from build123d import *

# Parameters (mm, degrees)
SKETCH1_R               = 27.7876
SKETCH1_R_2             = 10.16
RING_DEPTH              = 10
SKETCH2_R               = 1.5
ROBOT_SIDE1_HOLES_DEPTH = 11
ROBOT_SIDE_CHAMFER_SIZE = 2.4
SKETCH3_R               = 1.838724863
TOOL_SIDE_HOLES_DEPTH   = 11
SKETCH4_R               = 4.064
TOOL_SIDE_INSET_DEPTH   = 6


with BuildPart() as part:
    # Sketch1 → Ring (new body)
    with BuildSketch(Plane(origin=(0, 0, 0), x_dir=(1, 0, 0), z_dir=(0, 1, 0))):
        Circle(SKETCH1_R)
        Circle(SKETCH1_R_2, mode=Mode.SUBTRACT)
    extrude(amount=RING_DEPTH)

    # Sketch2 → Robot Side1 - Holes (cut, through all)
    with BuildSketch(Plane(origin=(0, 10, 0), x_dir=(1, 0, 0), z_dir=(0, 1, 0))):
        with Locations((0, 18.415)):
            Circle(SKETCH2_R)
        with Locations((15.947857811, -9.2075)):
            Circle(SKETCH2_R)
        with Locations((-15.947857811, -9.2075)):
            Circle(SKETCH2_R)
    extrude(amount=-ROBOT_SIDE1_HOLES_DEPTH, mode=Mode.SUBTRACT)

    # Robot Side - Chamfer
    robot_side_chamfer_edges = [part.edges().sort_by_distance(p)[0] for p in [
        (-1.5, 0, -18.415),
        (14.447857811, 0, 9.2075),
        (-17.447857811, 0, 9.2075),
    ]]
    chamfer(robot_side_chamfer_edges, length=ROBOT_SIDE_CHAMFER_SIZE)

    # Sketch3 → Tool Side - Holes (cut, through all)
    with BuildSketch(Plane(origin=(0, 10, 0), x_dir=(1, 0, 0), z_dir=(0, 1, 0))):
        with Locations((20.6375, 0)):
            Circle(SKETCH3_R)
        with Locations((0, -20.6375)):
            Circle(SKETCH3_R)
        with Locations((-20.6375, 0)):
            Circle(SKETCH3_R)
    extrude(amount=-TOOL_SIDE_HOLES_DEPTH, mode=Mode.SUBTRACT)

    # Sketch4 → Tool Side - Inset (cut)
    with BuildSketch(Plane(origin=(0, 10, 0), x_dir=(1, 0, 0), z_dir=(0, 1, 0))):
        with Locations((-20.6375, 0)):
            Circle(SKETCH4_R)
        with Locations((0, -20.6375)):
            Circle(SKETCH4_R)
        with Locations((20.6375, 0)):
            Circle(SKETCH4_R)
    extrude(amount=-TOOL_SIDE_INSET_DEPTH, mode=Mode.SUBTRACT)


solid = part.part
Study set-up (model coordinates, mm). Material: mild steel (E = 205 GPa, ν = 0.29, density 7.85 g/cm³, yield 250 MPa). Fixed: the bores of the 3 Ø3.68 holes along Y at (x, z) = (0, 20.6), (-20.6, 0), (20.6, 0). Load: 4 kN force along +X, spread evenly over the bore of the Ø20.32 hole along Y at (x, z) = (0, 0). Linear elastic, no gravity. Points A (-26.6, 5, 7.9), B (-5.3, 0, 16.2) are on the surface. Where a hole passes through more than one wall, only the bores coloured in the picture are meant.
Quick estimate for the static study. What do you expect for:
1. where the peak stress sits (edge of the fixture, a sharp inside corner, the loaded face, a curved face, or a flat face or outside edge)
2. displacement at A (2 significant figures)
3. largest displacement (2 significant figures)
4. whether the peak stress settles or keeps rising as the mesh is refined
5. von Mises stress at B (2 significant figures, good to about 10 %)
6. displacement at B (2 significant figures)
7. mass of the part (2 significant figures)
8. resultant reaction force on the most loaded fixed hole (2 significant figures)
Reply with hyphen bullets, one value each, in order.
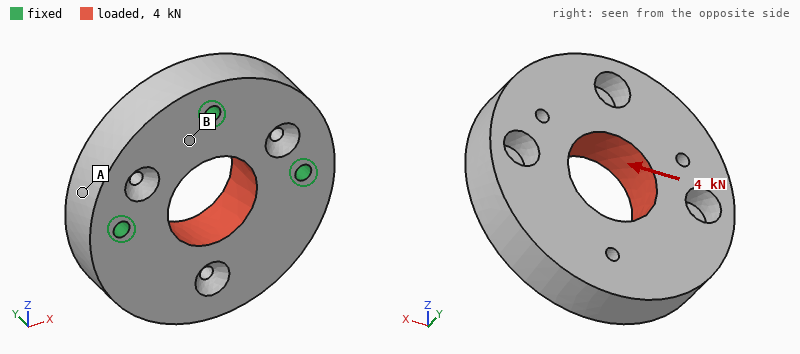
- edge of the fixture
- 1.3 µm
- 2.3 µm
- keeps rising
- 12 MPa
- 0.48 µm
- 150 g
- 1.6 kN
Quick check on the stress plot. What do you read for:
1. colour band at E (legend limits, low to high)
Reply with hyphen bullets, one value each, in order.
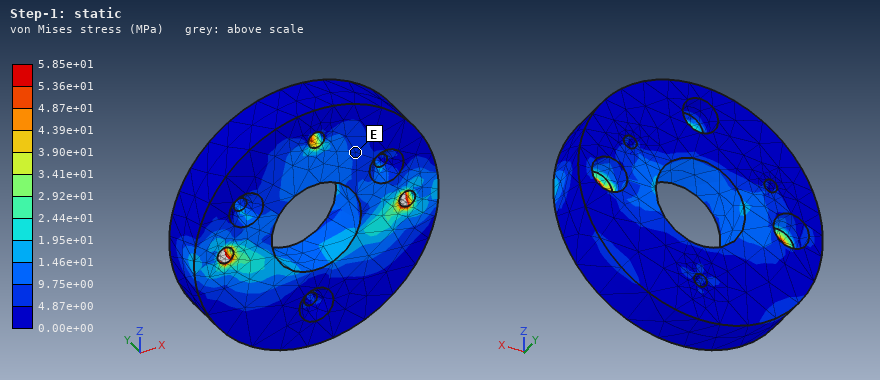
- 4.87e+00 to 9.75e+00 MPa
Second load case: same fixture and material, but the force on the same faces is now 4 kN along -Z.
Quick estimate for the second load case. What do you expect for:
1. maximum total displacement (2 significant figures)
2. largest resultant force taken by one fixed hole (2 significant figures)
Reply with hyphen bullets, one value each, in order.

- 6.6 µm
- 1.4 kN
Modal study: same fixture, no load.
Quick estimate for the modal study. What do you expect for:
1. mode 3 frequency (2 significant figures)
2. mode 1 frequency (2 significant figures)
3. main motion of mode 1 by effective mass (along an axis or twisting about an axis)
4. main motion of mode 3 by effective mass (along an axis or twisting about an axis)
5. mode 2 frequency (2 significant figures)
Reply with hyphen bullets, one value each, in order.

- 18 kHz
- 6000 Hz
- along Y
- along X
- 15 kHz
